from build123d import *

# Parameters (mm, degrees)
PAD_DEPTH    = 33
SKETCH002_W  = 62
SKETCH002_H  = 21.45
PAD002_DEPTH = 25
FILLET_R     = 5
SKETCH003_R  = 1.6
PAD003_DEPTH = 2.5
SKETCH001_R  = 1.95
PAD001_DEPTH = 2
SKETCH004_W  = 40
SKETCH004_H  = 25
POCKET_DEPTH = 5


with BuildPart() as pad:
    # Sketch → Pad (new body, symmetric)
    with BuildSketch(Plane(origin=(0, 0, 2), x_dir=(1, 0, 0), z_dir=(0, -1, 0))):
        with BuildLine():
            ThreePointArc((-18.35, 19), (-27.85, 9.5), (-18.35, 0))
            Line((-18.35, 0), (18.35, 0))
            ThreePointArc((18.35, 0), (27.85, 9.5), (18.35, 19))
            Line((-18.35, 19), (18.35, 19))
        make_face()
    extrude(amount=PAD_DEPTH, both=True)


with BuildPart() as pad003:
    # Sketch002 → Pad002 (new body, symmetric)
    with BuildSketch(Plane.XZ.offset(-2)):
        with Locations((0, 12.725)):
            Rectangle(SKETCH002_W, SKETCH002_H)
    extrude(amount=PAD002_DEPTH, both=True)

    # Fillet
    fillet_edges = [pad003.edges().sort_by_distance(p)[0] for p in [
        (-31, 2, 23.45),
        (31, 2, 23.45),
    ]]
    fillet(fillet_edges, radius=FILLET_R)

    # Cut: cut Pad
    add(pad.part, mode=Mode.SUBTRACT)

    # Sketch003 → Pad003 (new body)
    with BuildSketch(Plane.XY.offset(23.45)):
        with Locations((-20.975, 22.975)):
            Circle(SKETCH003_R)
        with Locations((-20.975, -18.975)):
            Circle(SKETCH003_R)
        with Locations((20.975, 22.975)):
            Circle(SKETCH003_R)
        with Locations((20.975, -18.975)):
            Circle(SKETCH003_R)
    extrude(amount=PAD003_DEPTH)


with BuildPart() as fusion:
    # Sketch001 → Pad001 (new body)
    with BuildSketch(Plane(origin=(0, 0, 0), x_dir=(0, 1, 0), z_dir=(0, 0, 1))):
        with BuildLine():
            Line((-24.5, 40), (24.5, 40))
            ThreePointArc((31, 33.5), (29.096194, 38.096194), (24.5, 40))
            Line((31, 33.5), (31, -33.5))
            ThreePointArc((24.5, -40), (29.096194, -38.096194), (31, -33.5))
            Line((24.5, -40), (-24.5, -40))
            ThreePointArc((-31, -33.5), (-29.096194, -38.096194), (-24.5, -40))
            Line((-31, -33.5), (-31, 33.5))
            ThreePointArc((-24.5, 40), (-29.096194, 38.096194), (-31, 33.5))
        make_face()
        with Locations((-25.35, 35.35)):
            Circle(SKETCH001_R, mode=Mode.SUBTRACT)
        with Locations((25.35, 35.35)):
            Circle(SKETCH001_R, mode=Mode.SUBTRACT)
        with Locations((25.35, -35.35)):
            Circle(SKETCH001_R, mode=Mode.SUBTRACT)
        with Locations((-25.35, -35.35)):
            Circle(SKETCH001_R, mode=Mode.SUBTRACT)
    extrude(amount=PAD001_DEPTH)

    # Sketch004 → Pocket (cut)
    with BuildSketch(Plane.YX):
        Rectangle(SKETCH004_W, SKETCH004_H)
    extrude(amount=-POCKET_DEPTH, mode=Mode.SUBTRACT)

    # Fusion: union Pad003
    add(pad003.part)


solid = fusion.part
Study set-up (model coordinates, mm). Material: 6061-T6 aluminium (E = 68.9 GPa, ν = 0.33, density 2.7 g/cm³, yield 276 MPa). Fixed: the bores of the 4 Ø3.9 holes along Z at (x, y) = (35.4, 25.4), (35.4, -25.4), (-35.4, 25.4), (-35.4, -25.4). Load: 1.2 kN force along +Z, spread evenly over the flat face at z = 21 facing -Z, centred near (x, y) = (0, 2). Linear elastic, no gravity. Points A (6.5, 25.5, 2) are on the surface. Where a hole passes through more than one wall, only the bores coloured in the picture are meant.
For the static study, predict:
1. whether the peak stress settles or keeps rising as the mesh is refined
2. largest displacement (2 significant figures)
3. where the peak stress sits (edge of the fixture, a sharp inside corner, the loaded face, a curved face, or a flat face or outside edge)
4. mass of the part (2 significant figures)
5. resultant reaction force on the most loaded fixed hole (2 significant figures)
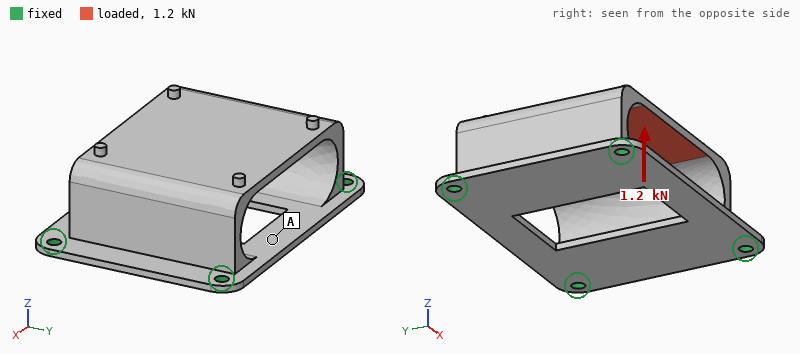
keeps rising
0.14 mm
edge of the fixture
67 g
450 N
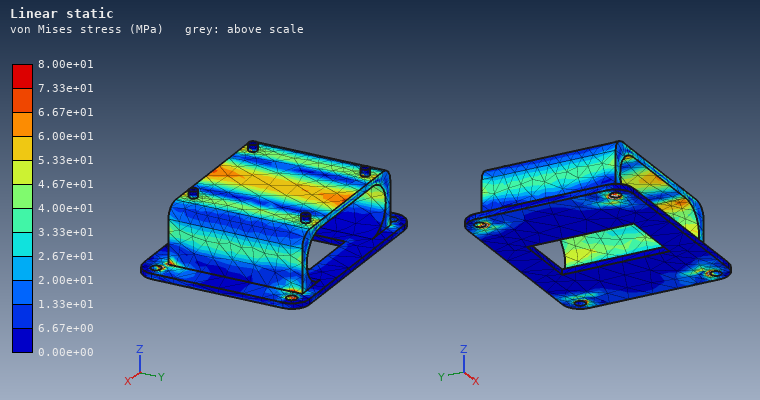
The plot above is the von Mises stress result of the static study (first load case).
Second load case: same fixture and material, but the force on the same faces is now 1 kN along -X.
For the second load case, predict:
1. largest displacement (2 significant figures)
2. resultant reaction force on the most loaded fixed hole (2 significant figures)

0.16 mm
330 N
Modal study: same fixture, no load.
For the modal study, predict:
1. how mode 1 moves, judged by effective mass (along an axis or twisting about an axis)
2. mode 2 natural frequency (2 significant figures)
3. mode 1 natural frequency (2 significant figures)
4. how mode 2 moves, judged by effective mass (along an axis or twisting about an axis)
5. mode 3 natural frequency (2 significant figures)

along X
4100 Hz
2300 Hz
along Z
4600 Hz
